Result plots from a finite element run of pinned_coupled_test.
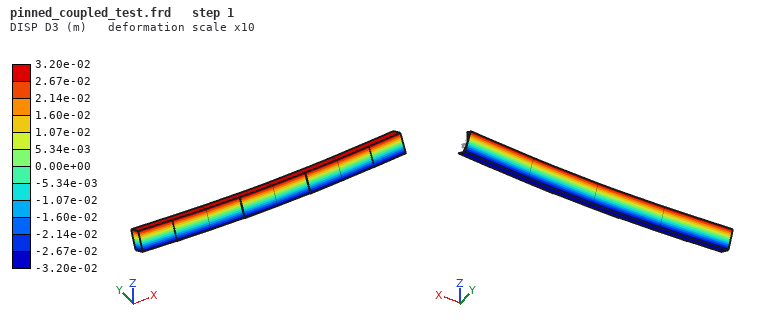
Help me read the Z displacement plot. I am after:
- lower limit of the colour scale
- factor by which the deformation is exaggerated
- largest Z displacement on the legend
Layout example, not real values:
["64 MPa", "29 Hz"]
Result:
["-3.20e-02 m", "10", "3.20e-02 m"]
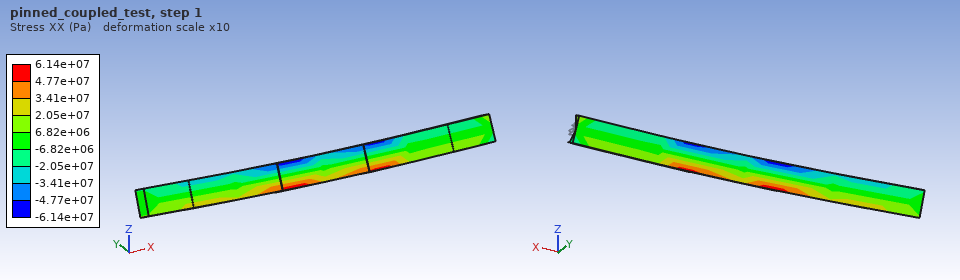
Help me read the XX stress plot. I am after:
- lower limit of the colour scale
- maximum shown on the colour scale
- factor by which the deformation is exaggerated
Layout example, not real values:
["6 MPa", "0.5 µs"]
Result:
["-6.14e+07 Pa", "6.14e+07 Pa", "10"]
